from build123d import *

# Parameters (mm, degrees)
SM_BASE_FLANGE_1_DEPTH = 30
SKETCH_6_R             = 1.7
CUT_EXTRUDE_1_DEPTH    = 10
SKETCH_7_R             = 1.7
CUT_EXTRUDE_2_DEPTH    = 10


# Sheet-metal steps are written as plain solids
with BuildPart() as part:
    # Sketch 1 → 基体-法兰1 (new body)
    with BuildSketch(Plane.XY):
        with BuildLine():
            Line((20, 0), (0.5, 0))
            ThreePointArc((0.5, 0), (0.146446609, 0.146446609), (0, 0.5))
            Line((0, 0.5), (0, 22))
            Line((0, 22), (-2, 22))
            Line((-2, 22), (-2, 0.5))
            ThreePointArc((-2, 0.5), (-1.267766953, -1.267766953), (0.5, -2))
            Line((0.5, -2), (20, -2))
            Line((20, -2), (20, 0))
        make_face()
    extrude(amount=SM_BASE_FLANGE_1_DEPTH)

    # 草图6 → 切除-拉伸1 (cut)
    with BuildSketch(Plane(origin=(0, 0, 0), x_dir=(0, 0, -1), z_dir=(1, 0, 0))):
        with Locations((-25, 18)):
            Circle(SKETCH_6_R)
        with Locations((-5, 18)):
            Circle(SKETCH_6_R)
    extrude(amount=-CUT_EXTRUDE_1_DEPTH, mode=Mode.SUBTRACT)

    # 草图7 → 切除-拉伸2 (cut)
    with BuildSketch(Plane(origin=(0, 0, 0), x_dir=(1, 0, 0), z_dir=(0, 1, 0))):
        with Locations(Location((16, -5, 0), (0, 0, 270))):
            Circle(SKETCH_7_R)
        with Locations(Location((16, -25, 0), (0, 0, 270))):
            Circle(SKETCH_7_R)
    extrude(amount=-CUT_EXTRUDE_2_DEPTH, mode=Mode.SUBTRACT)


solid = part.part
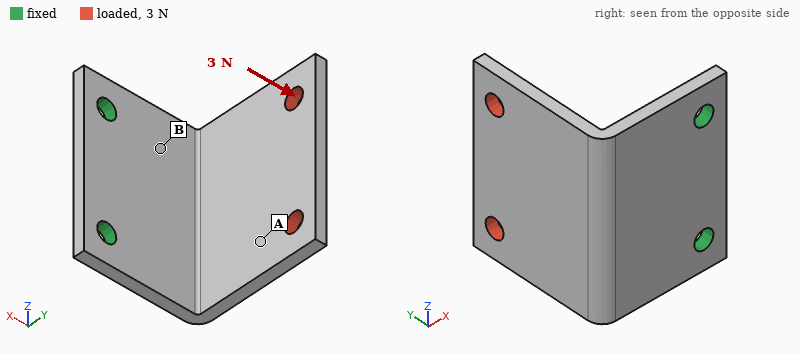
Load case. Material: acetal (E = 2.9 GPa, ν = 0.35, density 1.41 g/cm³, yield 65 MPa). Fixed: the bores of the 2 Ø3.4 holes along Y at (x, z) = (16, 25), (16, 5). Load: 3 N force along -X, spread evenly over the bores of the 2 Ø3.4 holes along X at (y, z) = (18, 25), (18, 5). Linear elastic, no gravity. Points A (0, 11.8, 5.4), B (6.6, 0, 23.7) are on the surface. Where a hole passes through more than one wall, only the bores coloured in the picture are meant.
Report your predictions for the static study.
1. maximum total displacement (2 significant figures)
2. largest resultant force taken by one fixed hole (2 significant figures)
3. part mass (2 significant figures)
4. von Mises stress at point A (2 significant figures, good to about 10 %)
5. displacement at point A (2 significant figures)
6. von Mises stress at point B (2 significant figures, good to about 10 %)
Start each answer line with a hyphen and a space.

- 0.51 mm
- 1.6 N
- 3.6 g
- 0.90 MPa
- 0.27 mm
- 2.6 MPa
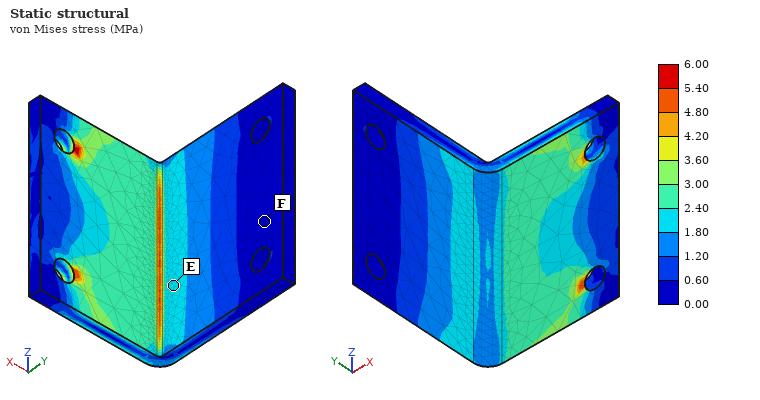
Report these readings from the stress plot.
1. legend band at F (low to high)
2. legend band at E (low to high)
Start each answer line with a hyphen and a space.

- 0.00 to 0.60 MPa
- 1.80 to 2.40 MPa
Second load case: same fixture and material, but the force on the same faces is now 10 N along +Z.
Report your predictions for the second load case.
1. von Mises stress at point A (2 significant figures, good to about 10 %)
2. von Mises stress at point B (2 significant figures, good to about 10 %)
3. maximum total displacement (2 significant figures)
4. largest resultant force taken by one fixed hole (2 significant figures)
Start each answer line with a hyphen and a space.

- 1.2 MPa
- 4.7 MPa
- 0.45 mm
- 13 N
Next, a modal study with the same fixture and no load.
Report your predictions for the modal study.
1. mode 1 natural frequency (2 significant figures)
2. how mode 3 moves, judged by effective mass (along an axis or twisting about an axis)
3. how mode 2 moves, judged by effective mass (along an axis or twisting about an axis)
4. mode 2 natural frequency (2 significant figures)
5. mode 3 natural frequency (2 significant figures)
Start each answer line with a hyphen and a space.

- 410 Hz
- along Y
- along Z
- 770 Hz
- 1200 Hz
